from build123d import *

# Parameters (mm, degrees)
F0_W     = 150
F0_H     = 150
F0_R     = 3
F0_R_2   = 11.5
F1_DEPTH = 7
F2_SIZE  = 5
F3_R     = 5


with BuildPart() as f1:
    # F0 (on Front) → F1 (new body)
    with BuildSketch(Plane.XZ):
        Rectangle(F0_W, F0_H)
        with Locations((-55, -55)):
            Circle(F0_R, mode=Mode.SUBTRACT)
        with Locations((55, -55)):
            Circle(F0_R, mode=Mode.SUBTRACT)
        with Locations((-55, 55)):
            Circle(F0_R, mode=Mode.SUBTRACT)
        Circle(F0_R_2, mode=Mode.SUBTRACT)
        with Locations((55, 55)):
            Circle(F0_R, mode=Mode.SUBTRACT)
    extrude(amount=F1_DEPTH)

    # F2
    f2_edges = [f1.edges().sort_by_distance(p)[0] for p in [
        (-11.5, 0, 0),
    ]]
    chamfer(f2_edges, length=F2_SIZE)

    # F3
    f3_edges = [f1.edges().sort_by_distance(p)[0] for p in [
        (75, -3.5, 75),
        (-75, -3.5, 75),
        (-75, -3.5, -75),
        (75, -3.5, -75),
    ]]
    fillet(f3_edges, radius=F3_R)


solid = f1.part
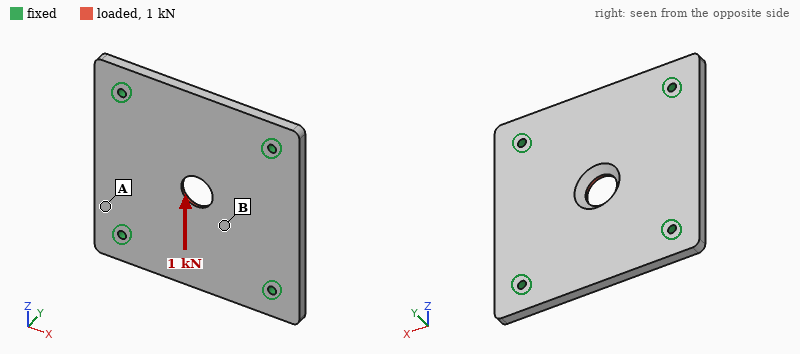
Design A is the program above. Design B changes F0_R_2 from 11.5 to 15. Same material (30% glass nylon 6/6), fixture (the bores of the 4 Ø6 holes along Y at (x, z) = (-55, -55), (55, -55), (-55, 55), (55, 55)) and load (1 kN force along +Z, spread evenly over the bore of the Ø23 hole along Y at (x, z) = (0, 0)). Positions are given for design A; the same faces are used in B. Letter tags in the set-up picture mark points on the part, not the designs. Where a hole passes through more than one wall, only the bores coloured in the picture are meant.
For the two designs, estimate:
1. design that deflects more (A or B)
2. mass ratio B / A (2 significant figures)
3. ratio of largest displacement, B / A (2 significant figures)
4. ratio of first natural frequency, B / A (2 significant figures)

A
0.98
0.90
1.0
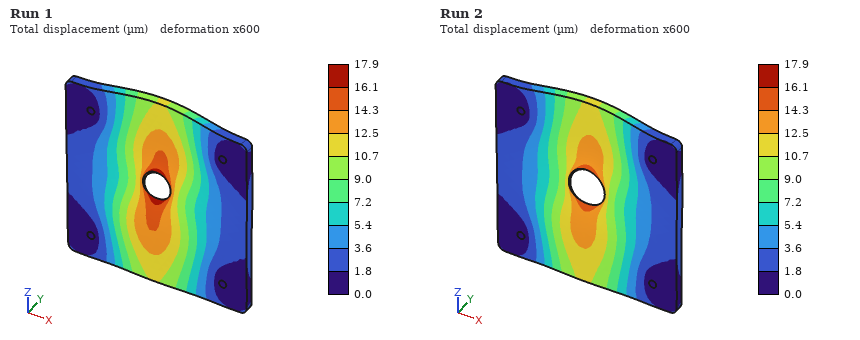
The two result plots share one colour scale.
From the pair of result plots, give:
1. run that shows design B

Run 2
